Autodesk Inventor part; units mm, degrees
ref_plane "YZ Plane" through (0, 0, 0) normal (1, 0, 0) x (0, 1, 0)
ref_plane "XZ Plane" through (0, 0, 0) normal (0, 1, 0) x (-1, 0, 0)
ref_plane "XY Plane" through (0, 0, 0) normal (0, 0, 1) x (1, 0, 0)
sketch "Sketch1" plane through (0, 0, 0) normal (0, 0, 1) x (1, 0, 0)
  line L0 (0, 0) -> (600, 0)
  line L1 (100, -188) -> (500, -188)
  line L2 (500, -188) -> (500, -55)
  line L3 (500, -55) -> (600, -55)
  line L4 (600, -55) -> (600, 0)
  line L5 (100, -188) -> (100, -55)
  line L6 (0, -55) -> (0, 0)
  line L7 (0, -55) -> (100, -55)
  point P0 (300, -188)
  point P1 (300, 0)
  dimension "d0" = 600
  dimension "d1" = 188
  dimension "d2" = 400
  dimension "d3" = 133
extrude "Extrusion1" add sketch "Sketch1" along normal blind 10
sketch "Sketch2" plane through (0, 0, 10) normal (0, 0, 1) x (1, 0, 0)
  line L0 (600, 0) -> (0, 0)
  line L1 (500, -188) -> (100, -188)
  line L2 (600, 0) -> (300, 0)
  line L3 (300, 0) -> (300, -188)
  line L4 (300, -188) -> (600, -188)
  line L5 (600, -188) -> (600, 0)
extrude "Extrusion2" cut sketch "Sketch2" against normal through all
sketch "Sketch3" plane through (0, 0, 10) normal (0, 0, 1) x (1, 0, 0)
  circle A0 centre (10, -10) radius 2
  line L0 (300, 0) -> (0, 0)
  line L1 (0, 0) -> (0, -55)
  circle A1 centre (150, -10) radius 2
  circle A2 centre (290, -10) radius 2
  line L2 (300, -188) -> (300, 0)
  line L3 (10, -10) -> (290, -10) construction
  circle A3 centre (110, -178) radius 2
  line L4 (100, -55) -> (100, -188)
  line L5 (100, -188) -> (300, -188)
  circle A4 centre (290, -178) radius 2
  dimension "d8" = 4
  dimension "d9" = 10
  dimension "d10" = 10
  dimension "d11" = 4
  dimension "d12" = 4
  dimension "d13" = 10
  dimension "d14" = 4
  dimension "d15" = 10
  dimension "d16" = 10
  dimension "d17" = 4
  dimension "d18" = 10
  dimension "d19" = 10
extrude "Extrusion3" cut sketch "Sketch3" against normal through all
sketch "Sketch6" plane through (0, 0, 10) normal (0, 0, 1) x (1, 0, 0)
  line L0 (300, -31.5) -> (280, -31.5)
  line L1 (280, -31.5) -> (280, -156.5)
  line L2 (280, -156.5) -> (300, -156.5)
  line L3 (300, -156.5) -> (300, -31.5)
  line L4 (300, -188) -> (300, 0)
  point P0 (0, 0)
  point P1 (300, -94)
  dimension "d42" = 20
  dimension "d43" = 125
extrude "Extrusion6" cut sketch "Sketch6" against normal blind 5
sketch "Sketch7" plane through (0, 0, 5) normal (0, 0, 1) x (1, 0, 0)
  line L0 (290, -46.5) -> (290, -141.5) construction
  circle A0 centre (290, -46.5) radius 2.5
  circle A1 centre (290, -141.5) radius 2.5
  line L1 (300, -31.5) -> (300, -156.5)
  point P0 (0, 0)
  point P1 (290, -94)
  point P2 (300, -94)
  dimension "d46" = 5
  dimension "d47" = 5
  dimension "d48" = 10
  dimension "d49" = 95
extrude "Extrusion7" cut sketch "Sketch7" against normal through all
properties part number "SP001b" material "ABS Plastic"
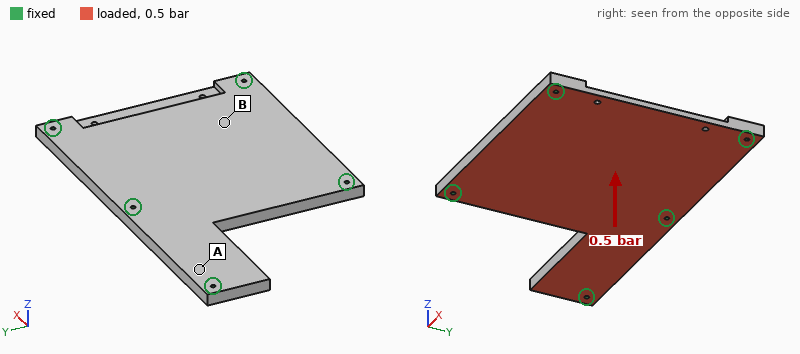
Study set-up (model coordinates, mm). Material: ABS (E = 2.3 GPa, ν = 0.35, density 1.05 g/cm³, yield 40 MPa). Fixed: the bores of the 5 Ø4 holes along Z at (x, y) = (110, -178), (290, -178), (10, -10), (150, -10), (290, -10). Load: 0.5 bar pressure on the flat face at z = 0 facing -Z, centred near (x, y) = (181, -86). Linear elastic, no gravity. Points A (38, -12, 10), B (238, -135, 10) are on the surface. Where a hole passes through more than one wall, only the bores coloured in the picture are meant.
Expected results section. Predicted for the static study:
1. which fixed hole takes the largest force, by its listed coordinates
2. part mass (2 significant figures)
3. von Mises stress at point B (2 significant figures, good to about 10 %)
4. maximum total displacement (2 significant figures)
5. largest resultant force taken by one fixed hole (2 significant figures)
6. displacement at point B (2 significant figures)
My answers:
(150, -10)
440 g
4.7 MPa
1.8 mm
670 N
1.6 mm
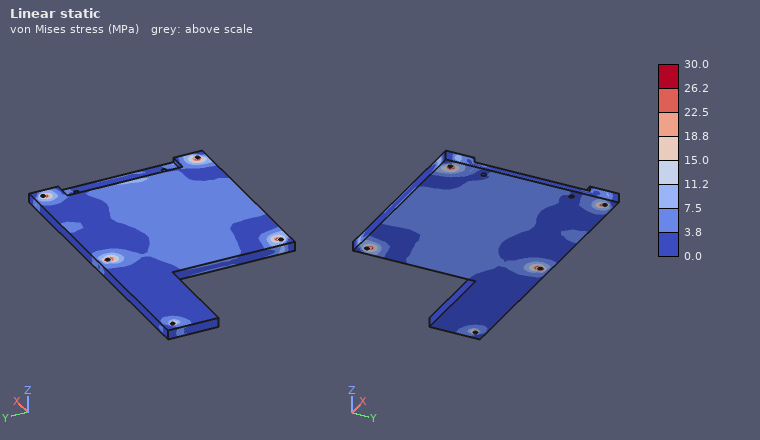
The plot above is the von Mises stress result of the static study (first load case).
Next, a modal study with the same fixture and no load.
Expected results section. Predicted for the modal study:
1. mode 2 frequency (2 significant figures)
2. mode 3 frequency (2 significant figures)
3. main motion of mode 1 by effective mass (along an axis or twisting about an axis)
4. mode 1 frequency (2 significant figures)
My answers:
450 Hz
510 Hz
along Z
310 Hz
